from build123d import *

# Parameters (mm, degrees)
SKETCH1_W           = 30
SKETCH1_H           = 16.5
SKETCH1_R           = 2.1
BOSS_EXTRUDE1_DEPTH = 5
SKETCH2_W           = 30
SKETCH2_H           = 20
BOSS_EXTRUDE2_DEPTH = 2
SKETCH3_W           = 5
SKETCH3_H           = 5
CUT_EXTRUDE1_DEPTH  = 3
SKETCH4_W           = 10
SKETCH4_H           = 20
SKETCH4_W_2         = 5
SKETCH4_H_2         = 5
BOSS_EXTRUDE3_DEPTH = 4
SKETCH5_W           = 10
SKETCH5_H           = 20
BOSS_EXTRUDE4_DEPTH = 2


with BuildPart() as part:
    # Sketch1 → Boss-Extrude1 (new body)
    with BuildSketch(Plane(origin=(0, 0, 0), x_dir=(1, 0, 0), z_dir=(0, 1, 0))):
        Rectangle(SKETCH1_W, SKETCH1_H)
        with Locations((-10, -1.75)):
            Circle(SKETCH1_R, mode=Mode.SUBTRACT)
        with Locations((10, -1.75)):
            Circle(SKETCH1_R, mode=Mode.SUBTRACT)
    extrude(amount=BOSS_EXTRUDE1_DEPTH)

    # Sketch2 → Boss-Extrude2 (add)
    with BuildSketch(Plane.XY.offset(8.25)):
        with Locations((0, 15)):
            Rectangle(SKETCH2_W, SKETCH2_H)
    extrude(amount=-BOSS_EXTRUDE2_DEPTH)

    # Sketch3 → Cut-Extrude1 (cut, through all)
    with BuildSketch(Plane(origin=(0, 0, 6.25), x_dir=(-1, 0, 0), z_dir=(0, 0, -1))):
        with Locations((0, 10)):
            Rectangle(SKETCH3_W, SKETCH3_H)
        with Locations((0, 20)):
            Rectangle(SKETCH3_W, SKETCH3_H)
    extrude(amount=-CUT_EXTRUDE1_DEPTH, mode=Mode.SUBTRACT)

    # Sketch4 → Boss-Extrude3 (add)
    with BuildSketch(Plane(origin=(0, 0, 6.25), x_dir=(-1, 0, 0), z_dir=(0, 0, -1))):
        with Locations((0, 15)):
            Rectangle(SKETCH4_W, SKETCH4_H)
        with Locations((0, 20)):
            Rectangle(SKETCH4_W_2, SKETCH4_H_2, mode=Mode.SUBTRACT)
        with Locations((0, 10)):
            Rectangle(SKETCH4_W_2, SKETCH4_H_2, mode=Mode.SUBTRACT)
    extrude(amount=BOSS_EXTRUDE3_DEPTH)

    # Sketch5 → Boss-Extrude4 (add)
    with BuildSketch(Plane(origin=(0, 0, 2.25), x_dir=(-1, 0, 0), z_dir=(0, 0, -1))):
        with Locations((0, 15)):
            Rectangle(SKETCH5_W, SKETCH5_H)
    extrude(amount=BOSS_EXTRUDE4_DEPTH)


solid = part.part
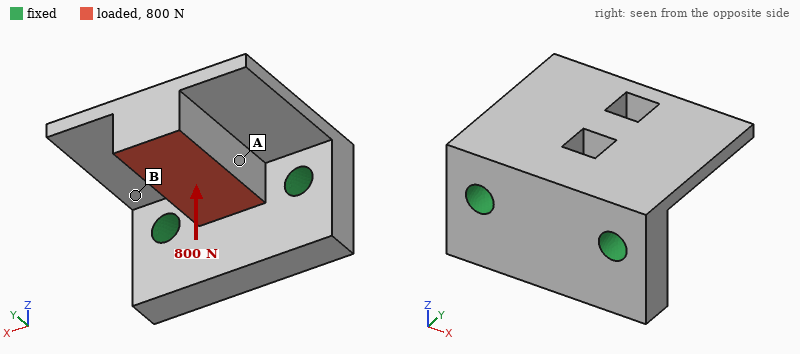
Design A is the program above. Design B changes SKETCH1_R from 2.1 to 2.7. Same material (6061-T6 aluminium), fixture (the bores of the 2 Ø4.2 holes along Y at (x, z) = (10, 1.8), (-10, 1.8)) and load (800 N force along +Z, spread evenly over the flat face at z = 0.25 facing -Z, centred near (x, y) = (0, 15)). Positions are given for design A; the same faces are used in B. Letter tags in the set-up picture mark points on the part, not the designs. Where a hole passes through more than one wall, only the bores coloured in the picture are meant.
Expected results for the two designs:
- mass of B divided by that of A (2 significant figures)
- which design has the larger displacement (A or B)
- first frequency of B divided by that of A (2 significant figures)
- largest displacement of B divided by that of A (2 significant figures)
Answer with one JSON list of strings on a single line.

["0.98", "A", "1.1", "0.89"]
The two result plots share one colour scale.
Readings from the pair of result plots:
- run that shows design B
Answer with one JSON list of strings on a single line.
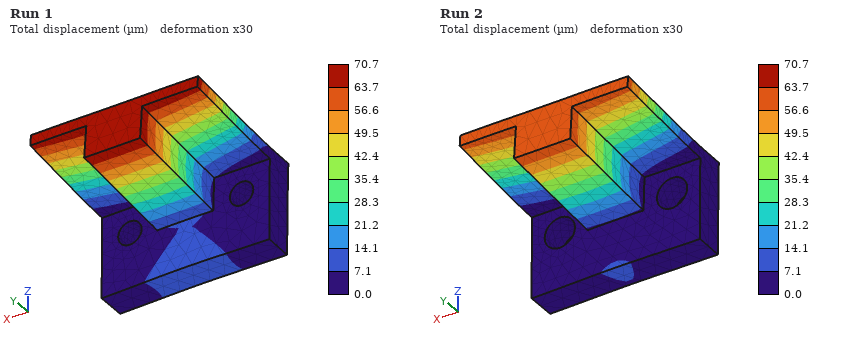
["Run 2"]
